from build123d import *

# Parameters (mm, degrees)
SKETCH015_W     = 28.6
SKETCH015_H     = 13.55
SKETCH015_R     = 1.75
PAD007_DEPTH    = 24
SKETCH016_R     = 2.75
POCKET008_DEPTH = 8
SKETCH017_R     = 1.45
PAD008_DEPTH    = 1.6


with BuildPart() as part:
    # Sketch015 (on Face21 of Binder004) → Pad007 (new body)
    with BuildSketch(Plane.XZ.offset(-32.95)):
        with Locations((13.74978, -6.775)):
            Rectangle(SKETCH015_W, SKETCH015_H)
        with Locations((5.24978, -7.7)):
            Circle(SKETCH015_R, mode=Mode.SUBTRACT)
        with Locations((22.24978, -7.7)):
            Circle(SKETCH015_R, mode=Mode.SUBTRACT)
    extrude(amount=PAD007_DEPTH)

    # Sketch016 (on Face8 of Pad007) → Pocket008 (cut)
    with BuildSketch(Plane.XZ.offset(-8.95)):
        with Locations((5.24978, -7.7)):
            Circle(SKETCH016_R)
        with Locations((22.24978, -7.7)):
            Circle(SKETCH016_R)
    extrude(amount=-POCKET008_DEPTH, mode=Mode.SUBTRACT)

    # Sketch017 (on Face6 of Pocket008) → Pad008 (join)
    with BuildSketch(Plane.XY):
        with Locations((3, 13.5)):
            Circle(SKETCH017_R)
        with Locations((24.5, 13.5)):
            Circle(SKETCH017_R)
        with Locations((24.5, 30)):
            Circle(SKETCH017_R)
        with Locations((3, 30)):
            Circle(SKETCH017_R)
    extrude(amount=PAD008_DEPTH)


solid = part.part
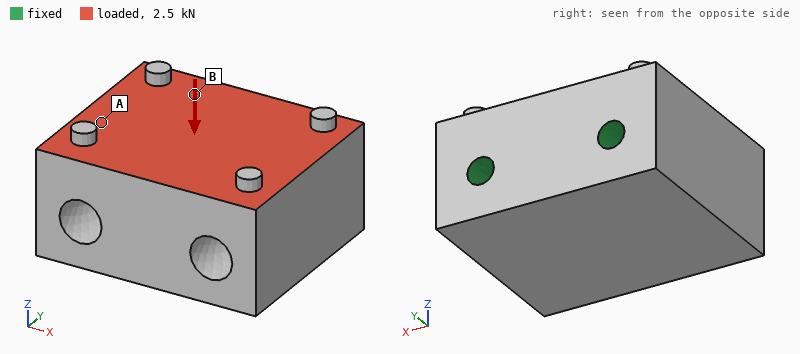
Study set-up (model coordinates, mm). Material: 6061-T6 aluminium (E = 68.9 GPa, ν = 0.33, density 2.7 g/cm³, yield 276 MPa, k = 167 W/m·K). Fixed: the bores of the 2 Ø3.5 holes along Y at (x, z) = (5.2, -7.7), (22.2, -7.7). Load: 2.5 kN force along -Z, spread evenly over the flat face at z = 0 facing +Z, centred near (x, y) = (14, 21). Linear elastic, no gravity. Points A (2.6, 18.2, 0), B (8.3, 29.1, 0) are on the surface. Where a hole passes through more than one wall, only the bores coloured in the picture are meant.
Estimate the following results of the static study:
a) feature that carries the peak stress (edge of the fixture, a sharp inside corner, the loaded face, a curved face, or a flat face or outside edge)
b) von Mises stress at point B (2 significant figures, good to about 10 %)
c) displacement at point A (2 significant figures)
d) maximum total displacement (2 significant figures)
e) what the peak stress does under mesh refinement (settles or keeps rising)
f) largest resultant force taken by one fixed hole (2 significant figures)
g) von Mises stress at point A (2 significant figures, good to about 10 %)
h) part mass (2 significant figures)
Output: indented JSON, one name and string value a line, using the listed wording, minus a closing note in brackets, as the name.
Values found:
{
  "feature that carries the peak stress": "edge of the fixture",
  "von Mises stress at point B": "4.2 MPa",
  "displacement at point A": "1.5 µm",
  "maximum total displacement": "3.8 µm",
  "what the peak stress does under mesh refinement": "keeps rising",
  "largest resultant force taken by one fixed hole": "1.3 kN",
  "von Mises stress at point A": "9.4 MPa",
  "part mass": "23 g"
}
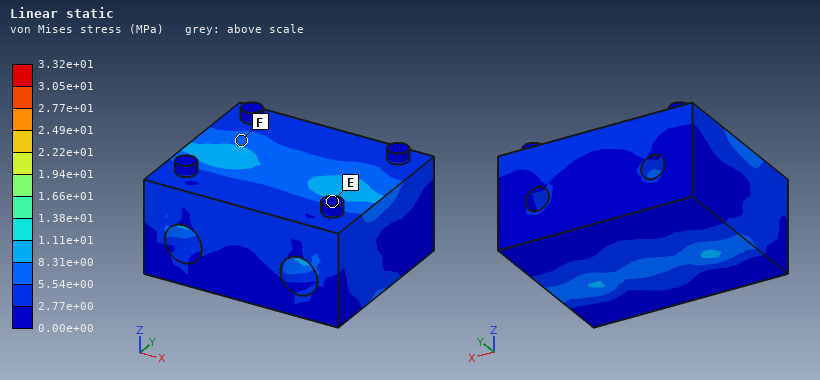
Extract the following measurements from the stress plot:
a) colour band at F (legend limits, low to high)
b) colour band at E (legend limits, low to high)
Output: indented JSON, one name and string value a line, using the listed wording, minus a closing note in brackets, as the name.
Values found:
{
  "colour band at F": "5.54e+00 to 8.31e+00 MPa",
  "colour band at E": "0.00e+00 to 2.77e+00 MPa"
}
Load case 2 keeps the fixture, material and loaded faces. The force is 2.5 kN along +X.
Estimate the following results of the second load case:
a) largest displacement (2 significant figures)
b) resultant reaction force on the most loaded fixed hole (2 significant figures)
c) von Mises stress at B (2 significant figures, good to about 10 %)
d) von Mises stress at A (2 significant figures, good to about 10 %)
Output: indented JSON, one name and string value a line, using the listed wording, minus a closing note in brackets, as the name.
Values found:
{
  "largest displacement": "4.3 µm",
  "resultant reaction force on the most loaded fixed hole": "1.6 kN",
  "von Mises stress at B": "7.6 MPa",
  "von Mises stress at A": "8.9 MPa"
}
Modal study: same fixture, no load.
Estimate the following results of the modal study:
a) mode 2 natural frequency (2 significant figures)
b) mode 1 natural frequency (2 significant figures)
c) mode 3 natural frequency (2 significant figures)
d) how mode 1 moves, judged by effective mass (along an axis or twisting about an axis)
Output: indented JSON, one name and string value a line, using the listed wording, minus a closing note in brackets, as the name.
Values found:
{
  "mode 2 natural frequency": "47 kHz",
  "mode 1 natural frequency": "34 kHz",
  "mode 3 natural frequency": "48 kHz",
  "how mode 1 moves, judged by effective mass": "along Z"
}
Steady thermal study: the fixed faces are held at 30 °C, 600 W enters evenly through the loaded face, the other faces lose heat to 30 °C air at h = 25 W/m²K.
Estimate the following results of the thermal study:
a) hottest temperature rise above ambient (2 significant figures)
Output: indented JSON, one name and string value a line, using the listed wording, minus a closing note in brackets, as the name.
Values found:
{
  "hottest temperature rise above ambient": "75 K"
}
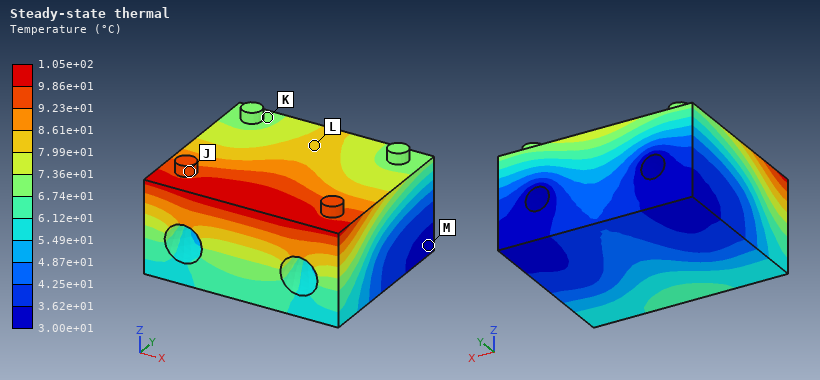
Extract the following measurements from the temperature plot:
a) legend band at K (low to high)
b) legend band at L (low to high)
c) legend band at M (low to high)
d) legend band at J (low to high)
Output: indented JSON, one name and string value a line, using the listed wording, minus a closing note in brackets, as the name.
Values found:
{
  "legend band at K": "6.74e+01 to 7.36e+01 °C",
  "legend band at L": "7.99e+01 to 8.61e+01 °C",
  "legend band at M": "3.00e+01 to 3.62e+01 °C",
  "legend band at J": "9.23e+01 to 9.86e+01 °C"
}
